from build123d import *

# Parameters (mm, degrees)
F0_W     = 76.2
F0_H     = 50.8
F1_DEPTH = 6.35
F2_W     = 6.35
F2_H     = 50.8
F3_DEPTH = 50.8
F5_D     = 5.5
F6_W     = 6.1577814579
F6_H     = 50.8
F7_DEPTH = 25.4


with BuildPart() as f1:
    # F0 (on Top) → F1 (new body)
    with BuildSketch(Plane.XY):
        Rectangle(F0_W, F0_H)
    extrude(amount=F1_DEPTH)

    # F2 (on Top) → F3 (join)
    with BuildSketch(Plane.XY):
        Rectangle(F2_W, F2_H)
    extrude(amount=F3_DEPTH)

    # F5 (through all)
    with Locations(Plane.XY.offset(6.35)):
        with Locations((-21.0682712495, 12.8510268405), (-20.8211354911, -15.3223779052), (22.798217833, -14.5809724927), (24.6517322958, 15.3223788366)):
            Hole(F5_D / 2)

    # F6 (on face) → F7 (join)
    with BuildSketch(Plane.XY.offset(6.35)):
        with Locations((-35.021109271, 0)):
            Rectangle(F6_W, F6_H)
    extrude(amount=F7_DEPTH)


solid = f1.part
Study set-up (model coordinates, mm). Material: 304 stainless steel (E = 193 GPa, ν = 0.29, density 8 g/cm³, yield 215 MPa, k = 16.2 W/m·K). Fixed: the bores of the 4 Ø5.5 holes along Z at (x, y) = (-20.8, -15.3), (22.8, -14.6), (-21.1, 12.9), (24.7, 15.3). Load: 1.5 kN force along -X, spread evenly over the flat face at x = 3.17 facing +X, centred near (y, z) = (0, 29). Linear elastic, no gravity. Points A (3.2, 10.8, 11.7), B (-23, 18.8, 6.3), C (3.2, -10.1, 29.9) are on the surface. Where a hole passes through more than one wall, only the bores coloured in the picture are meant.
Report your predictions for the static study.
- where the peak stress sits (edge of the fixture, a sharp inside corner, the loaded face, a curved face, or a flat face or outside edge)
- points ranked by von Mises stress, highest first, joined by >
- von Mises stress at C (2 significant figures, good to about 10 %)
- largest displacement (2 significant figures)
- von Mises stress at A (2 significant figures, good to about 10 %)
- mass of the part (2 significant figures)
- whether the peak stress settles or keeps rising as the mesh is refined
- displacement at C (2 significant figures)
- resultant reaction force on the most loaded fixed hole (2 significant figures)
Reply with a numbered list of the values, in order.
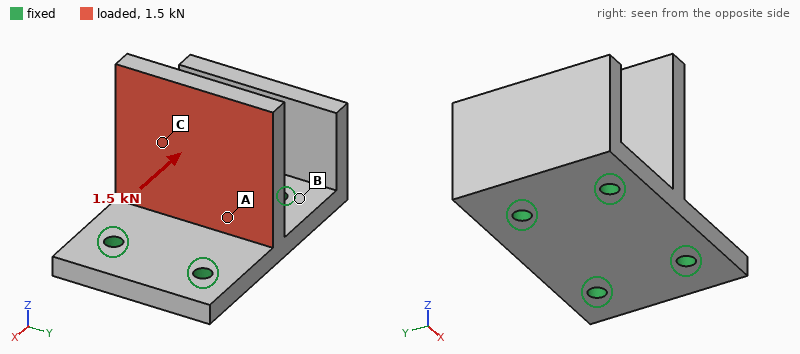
1. edge of the fixture
2. A > C > B
3. 21 MPa
4. 0.11 mm
5. 68 MPa
6. 370 g
7. keeps rising
8. 0.049 mm
9. 750 N
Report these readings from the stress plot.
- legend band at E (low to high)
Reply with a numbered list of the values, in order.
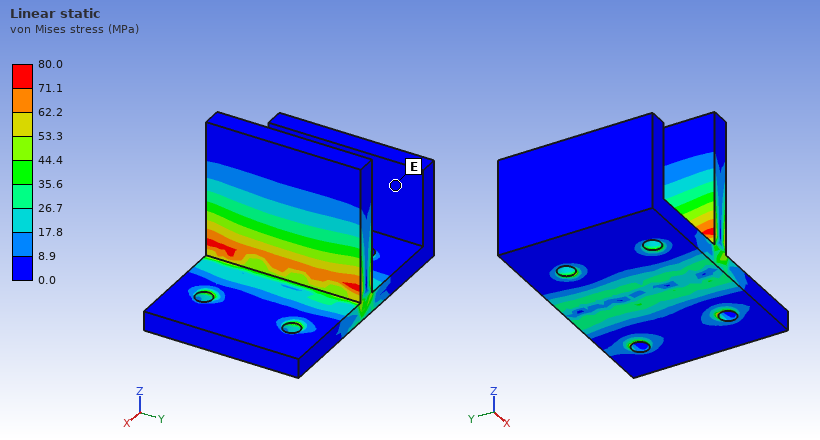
1. 0.0 to 8.9 MPa
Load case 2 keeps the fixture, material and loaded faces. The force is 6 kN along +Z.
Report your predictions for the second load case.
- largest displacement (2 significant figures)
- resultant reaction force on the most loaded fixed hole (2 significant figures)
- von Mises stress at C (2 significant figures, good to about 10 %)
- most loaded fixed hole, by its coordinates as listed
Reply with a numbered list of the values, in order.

1. 83 µm
2. 1.8 kN
3. 34 MPa
4. (22.8, -14.6)
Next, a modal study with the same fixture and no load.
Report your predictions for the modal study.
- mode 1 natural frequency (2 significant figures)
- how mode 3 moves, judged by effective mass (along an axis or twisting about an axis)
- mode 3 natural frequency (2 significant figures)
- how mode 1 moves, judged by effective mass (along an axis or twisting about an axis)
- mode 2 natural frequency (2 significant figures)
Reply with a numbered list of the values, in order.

1. 2200 Hz
2. along Y
3. 4400 Hz
4. along X
5. 3600 Hz
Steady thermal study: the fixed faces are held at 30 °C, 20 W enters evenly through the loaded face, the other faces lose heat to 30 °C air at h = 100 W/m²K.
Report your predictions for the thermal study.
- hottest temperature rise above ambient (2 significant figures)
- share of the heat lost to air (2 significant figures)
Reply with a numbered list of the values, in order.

1. 46 K
2. 74 %
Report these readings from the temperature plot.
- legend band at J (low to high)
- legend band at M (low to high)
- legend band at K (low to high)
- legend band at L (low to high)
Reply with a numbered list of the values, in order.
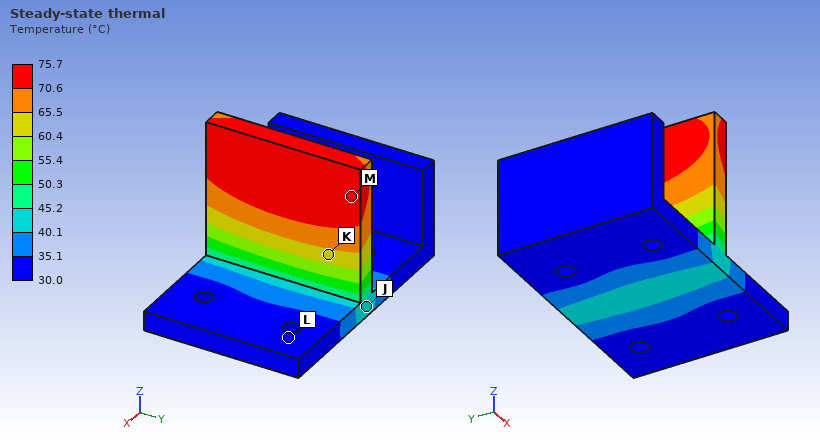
1. 40.1 to 45.2 °C
2. 70.6 to 75.7 °C
3. 60.4 to 65.5 °C
4. 30.0 to 35.1 °C
